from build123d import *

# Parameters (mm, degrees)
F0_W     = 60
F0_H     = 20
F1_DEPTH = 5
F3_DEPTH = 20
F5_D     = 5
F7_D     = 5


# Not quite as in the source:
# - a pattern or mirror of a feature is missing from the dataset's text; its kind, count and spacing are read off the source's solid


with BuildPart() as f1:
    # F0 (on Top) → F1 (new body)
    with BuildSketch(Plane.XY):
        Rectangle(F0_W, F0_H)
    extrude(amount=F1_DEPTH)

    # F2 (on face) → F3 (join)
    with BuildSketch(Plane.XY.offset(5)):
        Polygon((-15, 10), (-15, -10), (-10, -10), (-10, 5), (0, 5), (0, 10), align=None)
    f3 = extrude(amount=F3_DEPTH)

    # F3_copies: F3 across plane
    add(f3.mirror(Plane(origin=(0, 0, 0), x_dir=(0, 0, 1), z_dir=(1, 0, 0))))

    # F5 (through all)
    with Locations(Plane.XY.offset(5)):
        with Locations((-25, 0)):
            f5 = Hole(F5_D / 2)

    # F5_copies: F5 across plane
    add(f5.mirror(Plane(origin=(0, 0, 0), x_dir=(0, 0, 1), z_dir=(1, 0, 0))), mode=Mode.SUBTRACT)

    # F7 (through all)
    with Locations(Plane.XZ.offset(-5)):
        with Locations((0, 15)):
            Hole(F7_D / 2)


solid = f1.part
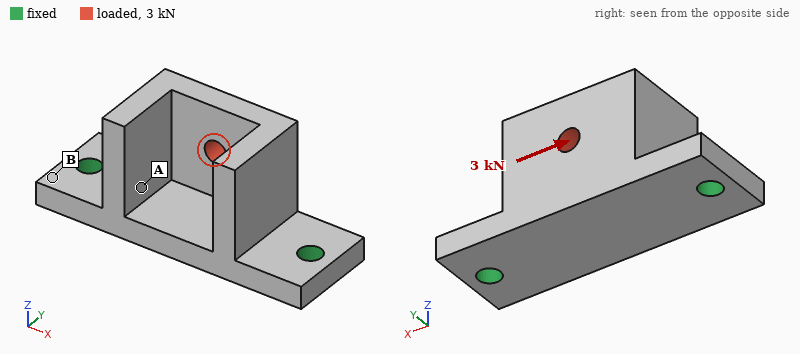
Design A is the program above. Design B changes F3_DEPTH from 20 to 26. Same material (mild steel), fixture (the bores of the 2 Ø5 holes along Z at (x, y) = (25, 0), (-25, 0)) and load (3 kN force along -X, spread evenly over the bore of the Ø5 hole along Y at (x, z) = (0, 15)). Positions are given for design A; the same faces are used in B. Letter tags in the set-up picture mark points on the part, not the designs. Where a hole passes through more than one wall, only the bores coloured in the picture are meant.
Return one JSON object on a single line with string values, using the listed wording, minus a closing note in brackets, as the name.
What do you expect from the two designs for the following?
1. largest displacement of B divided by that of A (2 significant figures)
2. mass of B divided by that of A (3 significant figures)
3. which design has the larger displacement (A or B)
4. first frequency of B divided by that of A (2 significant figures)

{"largest displacement of B divided by that of A": "1.1", "mass of B divided by that of A": "1.15", "which design has the larger displacement": "B", "first frequency of B divided by that of A": "0.74"}
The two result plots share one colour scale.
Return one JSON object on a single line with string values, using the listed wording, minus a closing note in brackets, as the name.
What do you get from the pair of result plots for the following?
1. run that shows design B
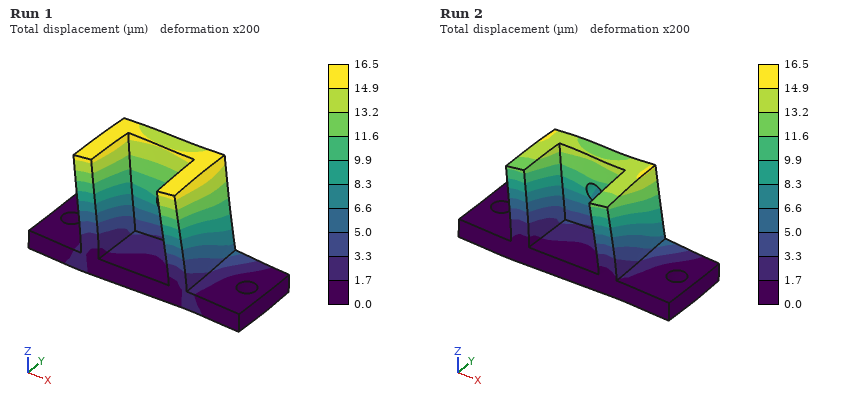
{"run that shows design B": "Run 1"}
